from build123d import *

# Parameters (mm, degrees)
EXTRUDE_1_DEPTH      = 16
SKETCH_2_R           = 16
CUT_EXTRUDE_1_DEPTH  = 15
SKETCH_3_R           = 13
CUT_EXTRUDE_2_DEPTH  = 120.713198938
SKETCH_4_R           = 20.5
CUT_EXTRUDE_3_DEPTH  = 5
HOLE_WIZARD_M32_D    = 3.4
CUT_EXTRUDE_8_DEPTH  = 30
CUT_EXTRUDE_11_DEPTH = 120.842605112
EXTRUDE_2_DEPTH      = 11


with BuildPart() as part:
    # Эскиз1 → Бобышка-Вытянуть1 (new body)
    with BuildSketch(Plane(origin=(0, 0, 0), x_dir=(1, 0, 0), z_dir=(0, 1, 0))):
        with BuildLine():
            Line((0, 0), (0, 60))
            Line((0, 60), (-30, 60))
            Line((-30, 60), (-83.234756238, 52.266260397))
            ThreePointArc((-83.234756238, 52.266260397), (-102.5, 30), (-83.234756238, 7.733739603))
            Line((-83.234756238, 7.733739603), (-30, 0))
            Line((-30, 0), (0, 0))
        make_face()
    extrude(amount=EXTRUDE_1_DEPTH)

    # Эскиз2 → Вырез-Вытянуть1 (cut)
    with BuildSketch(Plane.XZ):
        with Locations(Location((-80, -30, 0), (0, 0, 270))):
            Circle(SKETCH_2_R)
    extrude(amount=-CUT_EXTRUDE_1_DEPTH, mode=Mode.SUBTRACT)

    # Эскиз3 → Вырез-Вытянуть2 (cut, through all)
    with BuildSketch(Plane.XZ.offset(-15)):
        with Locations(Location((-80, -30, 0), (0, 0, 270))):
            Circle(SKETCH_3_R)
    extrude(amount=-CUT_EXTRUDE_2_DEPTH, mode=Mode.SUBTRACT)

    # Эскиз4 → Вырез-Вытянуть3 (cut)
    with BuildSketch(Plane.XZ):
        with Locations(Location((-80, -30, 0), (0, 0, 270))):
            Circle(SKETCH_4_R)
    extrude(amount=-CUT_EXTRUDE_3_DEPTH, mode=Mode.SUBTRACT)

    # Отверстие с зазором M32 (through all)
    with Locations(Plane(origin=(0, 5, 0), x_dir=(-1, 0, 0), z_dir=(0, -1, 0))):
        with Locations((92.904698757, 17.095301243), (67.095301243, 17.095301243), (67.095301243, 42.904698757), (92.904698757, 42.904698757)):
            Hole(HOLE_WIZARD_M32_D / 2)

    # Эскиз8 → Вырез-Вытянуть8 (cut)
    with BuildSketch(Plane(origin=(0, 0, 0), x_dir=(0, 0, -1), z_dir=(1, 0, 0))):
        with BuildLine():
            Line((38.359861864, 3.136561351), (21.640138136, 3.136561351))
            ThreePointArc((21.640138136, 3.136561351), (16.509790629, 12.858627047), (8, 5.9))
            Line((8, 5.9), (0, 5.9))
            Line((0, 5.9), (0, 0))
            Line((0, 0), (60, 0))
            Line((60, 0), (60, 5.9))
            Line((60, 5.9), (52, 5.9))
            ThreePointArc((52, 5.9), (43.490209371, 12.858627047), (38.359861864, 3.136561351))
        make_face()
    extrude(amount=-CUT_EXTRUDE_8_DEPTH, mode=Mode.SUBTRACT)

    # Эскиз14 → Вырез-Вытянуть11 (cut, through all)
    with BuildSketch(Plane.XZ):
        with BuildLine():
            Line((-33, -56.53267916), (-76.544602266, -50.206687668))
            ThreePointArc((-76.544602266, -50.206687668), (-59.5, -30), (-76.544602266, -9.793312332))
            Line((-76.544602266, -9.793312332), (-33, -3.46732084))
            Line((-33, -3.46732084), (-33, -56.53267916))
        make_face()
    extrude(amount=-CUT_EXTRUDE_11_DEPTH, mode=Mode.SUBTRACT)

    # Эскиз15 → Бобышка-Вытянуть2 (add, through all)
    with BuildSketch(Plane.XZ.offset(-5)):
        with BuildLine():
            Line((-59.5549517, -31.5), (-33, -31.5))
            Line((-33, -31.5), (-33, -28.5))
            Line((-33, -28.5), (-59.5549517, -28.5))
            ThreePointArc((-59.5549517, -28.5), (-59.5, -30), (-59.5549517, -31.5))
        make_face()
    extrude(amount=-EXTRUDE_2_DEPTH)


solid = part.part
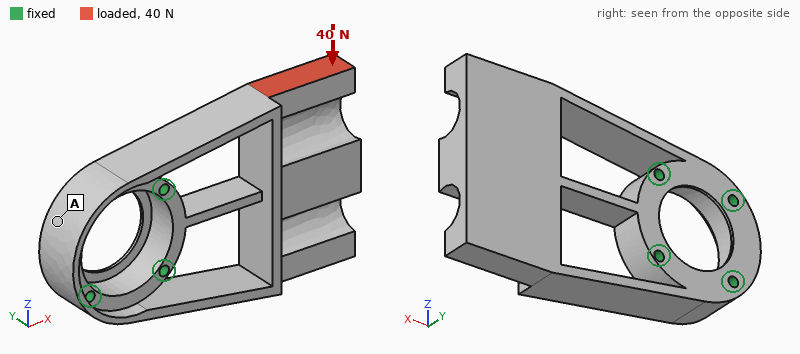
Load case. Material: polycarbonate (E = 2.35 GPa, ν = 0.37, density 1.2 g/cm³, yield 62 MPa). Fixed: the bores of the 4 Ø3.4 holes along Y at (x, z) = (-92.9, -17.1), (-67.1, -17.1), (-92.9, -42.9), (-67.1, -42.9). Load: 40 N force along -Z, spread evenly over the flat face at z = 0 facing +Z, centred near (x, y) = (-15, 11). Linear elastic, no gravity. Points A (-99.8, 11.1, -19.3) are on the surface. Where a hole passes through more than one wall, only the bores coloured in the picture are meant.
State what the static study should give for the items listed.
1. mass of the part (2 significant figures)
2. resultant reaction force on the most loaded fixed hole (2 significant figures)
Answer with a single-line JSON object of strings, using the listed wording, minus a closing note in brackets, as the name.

{"mass of the part": "37 g", "resultant reaction force on the most loaded fixed hole": "59 N"}
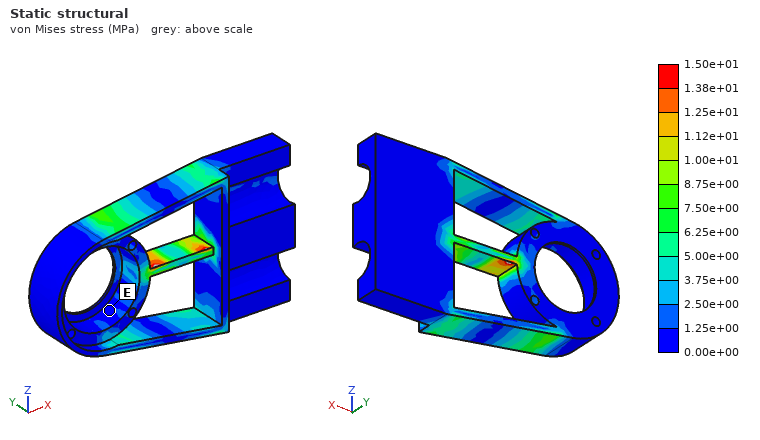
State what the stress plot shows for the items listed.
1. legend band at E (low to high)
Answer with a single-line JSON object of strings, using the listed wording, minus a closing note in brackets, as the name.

{"legend band at E": "0.00e+00 to 1.25e+00 MPa"}
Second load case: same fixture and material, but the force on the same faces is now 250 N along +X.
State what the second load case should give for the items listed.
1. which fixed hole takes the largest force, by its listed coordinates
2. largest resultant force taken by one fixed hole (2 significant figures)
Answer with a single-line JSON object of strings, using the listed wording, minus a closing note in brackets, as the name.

{"which fixed hole takes the largest force, by its listed coordinates": "(-67.1, -17.1)", "largest resultant force taken by one fixed hole": "200 N"}
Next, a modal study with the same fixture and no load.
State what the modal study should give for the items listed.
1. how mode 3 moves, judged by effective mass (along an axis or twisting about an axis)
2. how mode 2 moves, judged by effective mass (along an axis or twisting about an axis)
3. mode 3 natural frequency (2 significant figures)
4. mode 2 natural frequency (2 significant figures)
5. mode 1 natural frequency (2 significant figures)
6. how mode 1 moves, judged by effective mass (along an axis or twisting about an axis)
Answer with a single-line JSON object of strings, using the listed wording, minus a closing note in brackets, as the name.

{"how mode 3 moves, judged by effective mass": "twisting about X", "how mode 2 moves, judged by effective mass": "along Y", "mode 3 natural frequency": "520 Hz", "mode 2 natural frequency": "260 Hz", "mode 1 natural frequency": "200 Hz", "how mode 1 moves, judged by effective mass": "along Z"}
